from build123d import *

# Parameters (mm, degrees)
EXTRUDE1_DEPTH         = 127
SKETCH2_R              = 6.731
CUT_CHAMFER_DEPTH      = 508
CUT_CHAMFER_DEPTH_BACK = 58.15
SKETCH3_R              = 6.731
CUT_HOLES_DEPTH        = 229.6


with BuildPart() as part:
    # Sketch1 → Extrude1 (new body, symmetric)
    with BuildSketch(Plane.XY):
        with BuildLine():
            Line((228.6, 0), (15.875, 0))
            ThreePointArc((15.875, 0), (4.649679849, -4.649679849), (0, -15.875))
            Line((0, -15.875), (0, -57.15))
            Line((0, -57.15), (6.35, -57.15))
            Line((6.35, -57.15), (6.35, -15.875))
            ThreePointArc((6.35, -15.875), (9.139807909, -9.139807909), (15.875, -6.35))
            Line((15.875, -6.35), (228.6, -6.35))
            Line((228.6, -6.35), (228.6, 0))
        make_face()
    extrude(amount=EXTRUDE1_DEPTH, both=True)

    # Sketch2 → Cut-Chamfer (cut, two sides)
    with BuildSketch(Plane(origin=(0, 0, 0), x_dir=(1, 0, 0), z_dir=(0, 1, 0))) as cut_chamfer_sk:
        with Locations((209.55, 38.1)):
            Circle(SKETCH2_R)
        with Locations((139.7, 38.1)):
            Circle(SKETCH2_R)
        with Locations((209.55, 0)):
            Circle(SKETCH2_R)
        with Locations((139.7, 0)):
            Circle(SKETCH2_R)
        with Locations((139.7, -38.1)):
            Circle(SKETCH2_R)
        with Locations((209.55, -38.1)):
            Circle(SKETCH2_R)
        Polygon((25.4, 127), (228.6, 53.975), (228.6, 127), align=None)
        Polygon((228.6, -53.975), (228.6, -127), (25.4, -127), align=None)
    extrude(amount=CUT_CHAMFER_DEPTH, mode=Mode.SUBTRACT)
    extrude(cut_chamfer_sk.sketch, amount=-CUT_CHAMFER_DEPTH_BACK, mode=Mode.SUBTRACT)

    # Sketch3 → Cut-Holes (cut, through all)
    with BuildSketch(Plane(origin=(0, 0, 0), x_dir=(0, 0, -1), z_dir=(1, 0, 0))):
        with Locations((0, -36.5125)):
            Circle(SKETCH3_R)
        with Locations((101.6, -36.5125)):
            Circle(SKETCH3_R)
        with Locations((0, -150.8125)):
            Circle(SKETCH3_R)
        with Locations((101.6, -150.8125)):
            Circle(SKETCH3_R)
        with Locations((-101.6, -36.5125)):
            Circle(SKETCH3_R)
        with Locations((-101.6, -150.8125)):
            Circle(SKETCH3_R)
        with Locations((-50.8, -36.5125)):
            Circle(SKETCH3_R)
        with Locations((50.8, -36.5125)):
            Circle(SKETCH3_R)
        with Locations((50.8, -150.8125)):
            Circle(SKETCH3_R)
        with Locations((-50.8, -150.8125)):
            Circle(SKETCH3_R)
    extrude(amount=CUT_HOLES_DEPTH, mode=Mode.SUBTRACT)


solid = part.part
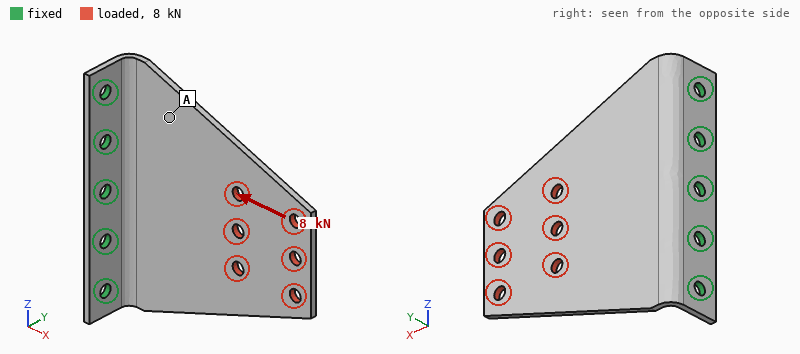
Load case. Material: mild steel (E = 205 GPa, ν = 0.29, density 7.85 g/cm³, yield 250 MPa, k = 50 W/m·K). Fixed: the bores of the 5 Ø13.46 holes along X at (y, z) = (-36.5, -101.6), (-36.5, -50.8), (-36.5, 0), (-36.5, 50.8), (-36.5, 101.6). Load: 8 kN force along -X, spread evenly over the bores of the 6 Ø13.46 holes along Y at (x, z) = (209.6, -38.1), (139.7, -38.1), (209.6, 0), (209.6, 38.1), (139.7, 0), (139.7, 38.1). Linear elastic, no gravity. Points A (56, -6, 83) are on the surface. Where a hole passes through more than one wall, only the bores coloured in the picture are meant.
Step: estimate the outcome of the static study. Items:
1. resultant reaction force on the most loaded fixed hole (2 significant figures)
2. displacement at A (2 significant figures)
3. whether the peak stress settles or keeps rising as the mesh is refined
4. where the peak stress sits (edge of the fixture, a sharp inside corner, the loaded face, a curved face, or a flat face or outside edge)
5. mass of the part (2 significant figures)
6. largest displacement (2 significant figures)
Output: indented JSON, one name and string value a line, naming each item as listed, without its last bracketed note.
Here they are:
{
  "resultant reaction force on the most loaded fixed hole": "1.7 kN",
  "displacement at A": "0.18 mm",
  "whether the peak stress settles or keeps rising as the mesh is refined": "keeps rising",
  "where the peak stress sits": "edge of the fixture",
  "mass of the part": "2.7 kg",
  "largest displacement": "0.74 mm"
}
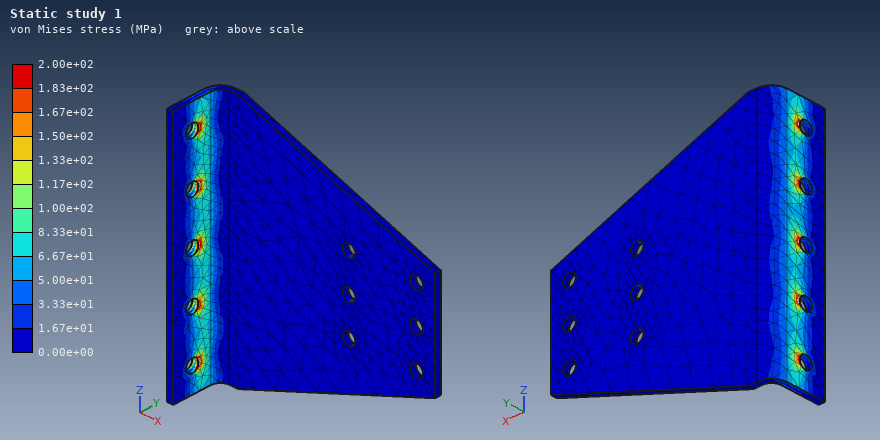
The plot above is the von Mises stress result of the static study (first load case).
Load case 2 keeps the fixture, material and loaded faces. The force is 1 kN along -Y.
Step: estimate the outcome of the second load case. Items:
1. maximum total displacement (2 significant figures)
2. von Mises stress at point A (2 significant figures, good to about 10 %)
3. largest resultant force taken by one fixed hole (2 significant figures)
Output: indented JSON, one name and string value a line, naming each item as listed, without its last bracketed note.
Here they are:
{
  "maximum total displacement": "3.4 mm",
  "von Mises stress at point A": "73 MPa",
  "largest resultant force taken by one fixed hole": "470 N"
}
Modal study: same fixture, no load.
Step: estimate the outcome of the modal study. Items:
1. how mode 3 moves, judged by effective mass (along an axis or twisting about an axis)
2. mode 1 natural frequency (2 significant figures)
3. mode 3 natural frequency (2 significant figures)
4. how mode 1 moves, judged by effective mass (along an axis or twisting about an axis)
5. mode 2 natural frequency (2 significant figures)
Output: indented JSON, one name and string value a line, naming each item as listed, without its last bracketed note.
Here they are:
{
  "how mode 3 moves, judged by effective mass": "along Y",
  "mode 1 natural frequency": "120 Hz",
  "mode 3 natural frequency": "590 Hz",
  "how mode 1 moves, judged by effective mass": "along Y",
  "mode 2 natural frequency": "390 Hz"
}
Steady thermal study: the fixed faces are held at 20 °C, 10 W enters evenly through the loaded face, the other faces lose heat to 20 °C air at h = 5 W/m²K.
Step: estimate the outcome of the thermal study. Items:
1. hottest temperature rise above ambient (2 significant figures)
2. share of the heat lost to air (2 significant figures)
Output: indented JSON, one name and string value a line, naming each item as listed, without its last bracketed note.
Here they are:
{
  "hottest temperature rise above ambient": "23 K",
  "share of the heat lost to air": "46 %"
}
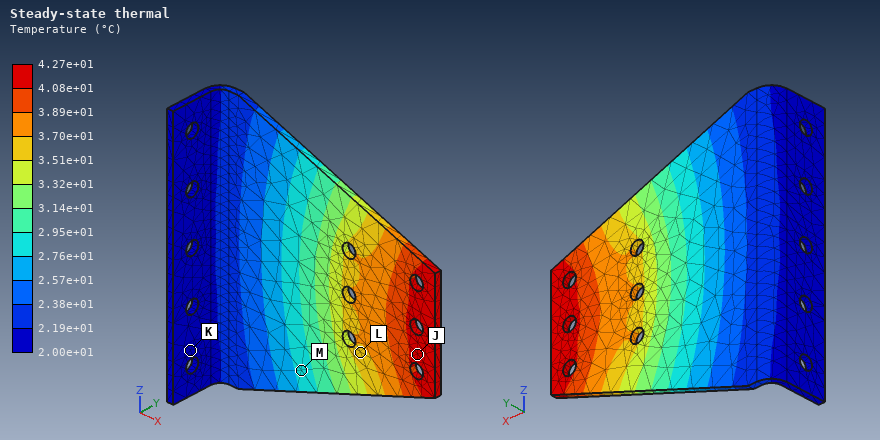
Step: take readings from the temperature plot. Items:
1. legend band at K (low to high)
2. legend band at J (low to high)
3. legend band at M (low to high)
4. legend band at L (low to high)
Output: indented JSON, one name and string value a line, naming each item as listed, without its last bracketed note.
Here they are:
{
  "legend band at K": "2.00e+01 to 2.19e+01 °C",
  "legend band at J": "4.08e+01 to 4.27e+01 °C",
  "legend band at M": "2.76e+01 to 2.95e+01 °C",
  "legend band at L": "3.51e+01 to 3.70e+01 °C"
}
